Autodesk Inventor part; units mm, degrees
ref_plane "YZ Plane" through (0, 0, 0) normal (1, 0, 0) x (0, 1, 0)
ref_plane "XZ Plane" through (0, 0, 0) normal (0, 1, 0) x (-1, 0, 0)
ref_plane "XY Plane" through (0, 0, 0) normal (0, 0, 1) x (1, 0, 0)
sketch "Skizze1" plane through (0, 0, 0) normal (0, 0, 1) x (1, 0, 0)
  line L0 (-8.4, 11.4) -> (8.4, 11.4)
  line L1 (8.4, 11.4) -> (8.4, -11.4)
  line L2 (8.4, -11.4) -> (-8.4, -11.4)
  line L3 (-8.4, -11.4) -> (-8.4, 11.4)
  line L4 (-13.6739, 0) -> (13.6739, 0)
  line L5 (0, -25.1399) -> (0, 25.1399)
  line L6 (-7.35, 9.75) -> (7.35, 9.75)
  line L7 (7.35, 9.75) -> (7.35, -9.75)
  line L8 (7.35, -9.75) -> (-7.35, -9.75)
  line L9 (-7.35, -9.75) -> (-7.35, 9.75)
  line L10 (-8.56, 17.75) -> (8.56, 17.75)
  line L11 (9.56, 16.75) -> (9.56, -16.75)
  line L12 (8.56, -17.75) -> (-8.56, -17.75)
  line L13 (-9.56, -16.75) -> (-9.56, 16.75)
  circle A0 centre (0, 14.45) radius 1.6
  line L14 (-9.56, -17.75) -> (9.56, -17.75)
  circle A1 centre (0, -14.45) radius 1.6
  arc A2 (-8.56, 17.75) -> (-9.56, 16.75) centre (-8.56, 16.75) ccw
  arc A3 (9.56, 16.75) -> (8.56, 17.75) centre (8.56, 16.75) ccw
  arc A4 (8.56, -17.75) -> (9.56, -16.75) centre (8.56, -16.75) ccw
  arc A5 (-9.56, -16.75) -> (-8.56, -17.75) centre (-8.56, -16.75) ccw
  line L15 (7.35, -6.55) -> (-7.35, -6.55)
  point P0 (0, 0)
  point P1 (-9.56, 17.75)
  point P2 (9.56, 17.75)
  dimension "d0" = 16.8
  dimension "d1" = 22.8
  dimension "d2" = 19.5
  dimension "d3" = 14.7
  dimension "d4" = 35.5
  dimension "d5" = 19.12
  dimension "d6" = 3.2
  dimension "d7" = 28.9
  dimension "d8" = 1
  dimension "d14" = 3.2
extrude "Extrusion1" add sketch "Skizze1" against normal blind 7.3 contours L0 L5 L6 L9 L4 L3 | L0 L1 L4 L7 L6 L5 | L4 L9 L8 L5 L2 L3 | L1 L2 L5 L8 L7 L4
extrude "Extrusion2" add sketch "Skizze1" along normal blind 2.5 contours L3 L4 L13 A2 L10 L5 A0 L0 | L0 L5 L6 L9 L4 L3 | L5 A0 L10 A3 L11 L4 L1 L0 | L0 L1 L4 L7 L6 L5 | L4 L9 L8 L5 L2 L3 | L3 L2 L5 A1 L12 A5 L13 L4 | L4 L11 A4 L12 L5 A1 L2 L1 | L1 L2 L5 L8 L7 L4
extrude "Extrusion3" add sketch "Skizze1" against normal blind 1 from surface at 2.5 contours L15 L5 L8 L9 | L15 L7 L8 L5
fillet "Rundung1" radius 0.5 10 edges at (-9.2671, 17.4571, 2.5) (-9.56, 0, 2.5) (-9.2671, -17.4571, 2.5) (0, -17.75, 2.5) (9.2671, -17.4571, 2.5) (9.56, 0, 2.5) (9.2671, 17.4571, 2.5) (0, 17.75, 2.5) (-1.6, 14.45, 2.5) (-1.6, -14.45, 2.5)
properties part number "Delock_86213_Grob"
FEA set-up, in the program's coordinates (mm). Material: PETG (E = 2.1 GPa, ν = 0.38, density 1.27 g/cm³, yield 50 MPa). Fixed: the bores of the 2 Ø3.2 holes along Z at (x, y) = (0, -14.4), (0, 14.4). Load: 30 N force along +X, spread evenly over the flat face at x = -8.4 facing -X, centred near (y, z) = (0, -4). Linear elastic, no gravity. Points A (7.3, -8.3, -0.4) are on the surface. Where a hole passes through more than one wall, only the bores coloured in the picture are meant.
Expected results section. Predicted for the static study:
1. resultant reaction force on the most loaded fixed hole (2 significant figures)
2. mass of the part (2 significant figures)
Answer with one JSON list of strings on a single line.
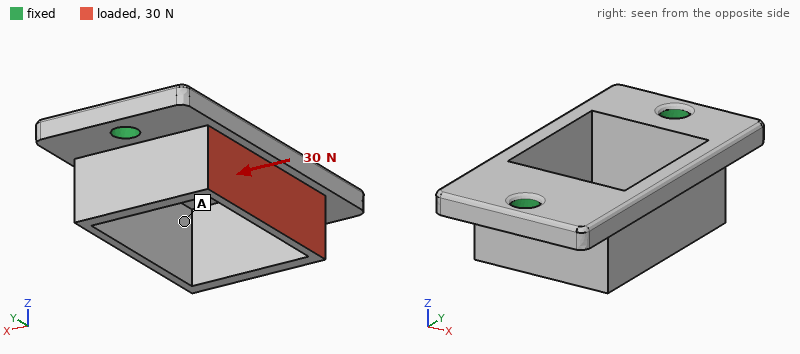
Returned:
["17 N", "2.1 g"]
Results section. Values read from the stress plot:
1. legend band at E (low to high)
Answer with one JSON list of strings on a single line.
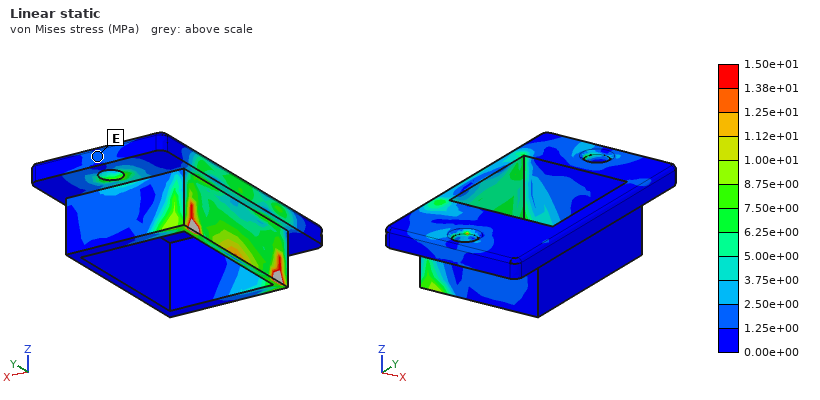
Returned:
["1.25e+00 to 2.50e+00 MPa"]
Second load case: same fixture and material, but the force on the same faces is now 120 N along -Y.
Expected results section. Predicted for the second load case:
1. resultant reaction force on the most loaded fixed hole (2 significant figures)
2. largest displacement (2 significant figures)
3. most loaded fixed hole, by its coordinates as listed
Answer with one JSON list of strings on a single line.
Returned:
["69 N", "0.21 mm", "(0, -14.4)"]
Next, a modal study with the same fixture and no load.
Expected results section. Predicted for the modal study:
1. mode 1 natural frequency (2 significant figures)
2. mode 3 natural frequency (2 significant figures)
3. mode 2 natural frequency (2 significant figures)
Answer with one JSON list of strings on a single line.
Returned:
["2800 Hz", "4200 Hz", "4000 Hz"]
